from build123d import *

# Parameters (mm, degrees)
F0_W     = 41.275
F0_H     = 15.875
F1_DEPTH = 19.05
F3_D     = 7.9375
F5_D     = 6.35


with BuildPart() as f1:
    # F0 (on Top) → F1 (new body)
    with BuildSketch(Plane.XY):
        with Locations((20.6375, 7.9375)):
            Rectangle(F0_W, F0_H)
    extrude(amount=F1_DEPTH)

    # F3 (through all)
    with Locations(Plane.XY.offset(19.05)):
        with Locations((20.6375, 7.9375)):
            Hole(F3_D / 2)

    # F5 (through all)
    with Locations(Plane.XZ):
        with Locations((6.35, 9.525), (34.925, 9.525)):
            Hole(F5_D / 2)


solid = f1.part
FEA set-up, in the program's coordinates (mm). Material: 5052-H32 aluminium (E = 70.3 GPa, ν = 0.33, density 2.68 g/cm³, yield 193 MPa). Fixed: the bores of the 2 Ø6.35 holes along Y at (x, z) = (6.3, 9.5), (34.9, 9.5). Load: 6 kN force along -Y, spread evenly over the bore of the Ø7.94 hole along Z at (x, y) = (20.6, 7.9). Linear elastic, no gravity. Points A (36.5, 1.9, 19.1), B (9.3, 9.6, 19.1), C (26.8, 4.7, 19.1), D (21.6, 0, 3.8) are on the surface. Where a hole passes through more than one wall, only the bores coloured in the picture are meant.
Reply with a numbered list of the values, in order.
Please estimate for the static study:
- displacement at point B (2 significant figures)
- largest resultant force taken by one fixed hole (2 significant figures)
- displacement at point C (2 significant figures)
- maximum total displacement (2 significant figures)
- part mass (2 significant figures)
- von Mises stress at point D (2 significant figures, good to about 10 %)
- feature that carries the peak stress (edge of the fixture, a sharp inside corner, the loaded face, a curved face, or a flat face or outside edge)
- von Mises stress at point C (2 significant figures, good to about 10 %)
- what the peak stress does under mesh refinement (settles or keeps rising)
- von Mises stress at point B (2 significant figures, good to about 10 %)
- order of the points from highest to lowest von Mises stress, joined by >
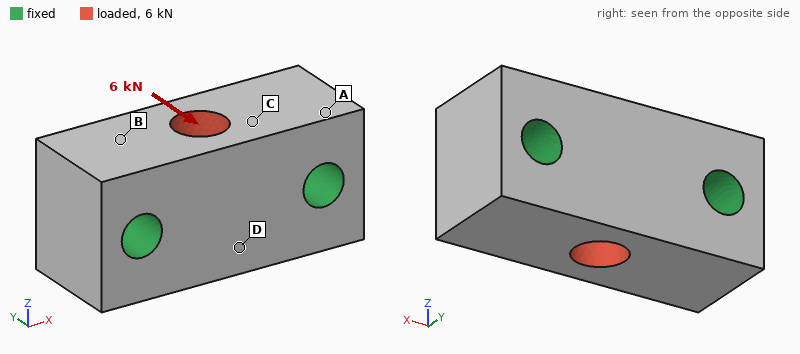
1. 1.7 µm
2. 3.0 kN
3. 4.3 µm
4. 7.4 µm
5. 28 g
6. 28 MPa
7. edge of the fixture
8. 19 MPa
9. keeps rising
10. 11 MPa
11. D > C > B > A
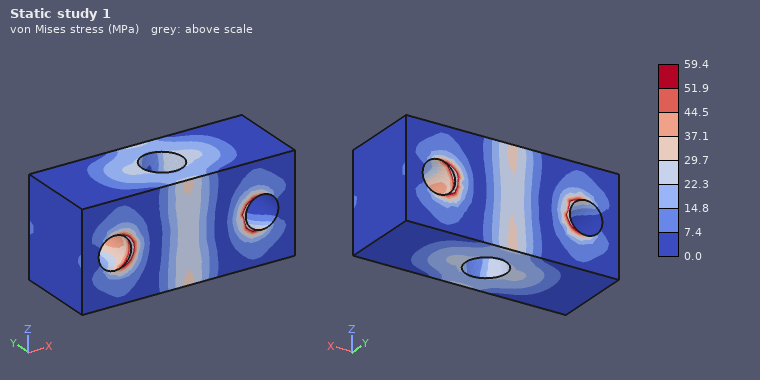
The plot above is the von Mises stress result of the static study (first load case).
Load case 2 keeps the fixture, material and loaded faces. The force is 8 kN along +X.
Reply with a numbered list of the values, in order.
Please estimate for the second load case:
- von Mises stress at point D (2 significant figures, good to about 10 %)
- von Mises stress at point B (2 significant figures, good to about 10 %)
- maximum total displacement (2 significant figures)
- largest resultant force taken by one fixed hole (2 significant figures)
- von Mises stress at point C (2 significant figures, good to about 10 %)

1. 4.5 MPa
2. 6.8 MPa
3. 3.2 µm
4. 4.0 kN
5. 14 MPa
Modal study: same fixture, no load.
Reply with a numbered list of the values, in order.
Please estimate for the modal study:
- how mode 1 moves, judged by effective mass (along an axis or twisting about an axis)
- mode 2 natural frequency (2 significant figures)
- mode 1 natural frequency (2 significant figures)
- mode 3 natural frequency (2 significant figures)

1. along Z
2. 53 kHz
3. 48 kHz
4. 54 kHz
